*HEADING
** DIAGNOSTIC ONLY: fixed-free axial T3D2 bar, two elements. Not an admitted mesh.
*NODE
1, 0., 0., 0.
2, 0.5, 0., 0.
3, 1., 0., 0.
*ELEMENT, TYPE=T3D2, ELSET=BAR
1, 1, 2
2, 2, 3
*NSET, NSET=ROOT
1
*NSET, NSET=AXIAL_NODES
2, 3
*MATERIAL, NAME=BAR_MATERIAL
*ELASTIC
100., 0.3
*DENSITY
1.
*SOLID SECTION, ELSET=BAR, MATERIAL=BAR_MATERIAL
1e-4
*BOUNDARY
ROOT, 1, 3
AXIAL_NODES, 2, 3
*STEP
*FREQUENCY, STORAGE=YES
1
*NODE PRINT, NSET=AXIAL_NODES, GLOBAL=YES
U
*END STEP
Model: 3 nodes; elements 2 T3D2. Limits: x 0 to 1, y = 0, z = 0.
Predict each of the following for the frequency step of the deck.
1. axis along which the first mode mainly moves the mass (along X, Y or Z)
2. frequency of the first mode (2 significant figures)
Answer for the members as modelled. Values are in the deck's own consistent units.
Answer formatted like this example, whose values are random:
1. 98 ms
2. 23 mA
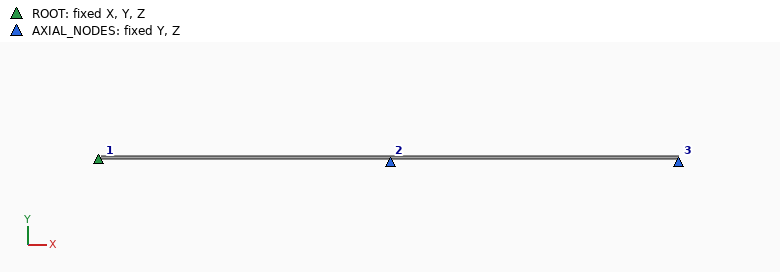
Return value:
1. along X
2. 2.6 cycles per unit time
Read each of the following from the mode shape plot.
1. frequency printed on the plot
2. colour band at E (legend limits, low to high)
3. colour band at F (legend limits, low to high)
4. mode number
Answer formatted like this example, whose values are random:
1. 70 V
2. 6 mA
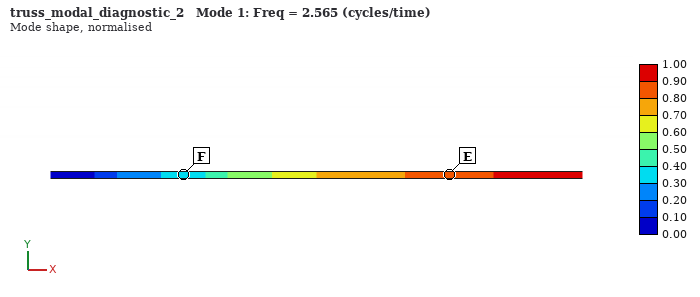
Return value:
1. 2.565
2. 0.80 to 0.90
3. 0.30 to 0.40
4. 1
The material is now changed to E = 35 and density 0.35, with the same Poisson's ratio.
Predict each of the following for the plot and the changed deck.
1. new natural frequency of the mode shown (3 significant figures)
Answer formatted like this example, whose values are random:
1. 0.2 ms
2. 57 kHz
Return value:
1. 2.56
